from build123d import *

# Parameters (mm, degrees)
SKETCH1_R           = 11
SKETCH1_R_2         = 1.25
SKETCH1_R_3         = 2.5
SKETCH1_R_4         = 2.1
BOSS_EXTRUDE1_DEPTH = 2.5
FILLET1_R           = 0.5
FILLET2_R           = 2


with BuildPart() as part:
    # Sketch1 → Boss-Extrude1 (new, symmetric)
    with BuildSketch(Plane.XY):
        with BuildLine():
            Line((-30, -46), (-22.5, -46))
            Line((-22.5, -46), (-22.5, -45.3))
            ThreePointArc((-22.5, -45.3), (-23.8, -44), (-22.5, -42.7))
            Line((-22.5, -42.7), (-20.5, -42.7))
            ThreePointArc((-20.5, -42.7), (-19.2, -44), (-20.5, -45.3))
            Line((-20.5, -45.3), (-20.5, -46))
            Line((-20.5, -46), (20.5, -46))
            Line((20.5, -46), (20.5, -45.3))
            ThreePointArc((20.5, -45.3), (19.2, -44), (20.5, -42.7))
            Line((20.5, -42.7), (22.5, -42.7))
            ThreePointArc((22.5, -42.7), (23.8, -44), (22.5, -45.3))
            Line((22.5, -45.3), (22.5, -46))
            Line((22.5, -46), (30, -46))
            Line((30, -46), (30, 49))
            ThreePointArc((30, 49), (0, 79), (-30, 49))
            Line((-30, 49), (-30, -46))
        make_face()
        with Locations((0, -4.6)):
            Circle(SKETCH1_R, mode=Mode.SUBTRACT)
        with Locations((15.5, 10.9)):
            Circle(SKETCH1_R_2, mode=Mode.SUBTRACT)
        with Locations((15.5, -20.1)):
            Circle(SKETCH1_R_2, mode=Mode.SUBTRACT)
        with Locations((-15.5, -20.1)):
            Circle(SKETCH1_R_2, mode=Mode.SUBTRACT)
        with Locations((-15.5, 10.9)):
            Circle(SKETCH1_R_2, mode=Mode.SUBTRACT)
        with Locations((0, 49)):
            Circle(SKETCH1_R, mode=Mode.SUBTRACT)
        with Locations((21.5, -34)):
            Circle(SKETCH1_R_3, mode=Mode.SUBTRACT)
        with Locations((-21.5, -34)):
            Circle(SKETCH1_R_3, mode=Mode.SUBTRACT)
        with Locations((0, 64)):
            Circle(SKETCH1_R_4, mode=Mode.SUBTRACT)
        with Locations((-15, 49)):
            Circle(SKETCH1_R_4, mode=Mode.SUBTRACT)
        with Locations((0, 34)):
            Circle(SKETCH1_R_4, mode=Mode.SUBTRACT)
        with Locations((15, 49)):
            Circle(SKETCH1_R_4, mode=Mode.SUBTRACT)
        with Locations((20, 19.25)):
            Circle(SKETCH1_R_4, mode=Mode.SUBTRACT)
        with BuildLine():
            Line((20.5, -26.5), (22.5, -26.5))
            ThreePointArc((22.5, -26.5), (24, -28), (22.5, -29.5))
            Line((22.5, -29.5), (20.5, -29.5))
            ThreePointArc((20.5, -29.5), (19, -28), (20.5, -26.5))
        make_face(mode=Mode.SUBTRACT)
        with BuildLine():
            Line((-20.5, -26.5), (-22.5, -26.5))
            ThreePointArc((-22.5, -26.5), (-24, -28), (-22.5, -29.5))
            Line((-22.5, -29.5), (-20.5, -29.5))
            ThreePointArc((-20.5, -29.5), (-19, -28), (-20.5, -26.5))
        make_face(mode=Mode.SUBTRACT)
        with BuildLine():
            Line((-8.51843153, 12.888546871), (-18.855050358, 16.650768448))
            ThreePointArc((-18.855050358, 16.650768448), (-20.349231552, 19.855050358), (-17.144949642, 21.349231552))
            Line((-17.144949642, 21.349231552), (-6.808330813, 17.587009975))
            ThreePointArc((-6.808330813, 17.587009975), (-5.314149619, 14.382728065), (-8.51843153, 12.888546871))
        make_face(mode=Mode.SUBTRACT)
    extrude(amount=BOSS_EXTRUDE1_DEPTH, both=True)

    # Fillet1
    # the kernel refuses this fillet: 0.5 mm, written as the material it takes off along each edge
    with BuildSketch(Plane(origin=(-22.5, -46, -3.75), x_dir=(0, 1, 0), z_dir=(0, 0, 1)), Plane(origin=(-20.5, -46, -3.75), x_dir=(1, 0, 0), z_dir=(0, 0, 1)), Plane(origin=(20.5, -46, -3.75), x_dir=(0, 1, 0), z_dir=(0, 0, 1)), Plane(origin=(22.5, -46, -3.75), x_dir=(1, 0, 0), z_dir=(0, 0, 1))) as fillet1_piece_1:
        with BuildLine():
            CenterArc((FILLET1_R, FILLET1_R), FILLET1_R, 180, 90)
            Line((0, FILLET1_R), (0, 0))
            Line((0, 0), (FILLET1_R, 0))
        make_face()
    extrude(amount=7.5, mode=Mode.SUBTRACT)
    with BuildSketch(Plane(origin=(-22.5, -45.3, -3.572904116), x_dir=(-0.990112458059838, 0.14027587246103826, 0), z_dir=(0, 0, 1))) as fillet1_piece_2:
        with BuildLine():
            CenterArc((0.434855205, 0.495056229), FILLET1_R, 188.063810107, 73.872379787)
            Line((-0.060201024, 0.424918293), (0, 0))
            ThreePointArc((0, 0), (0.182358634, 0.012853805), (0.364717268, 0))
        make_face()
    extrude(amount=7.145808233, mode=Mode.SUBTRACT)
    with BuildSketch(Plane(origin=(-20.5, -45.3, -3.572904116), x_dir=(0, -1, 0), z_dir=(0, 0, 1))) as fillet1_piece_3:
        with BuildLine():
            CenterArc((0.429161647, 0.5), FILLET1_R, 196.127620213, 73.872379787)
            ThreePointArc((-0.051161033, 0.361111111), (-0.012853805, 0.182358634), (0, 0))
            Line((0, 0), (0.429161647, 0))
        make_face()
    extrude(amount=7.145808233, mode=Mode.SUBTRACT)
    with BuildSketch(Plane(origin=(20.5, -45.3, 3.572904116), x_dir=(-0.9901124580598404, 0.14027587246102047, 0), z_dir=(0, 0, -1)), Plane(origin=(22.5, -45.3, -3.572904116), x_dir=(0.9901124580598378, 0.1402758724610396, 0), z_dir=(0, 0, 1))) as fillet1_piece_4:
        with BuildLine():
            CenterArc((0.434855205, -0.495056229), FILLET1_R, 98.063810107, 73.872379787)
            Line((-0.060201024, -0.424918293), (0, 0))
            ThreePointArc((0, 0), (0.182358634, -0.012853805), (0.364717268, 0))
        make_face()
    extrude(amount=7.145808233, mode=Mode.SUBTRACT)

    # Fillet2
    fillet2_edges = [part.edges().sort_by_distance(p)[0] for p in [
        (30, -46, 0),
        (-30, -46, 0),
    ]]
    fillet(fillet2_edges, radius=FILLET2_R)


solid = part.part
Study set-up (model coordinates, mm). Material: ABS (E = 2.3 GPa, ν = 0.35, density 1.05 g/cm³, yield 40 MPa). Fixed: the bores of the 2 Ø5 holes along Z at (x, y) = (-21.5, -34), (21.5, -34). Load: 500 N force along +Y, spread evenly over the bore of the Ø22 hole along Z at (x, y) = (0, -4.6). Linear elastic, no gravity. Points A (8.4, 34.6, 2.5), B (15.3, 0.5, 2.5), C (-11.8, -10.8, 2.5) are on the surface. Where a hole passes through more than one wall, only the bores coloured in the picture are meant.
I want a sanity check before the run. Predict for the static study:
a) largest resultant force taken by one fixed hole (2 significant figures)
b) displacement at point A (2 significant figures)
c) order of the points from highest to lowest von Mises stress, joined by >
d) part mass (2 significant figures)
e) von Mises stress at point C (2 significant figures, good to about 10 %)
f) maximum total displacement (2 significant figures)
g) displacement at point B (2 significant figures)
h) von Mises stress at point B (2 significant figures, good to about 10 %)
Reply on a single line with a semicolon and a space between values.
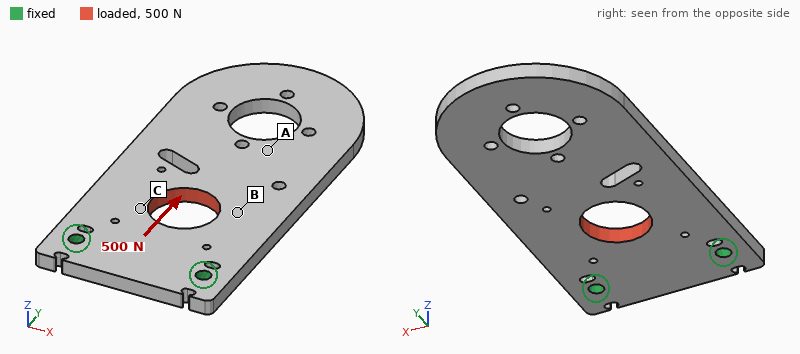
250 N; 44 µm; C > B > A; 32 g; 2.4 MPa; 56 µm; 39 µm; 1.3 MPa
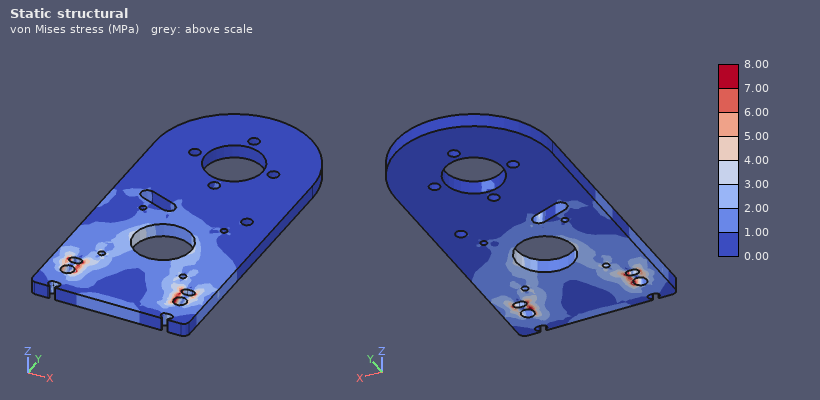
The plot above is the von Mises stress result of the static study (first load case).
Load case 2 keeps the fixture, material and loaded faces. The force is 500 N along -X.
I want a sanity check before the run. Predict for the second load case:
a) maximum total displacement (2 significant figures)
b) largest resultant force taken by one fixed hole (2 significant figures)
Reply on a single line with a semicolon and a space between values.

0.31 mm; 400 N
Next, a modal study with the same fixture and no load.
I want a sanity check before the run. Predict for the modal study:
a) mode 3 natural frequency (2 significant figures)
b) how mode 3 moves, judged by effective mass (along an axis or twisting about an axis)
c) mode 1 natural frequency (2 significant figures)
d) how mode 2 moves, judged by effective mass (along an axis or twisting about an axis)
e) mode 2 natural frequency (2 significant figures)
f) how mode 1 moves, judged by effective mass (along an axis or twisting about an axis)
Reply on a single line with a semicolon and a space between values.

560 Hz; along Z; 95 Hz; twisting about Y; 380 Hz; along Z
